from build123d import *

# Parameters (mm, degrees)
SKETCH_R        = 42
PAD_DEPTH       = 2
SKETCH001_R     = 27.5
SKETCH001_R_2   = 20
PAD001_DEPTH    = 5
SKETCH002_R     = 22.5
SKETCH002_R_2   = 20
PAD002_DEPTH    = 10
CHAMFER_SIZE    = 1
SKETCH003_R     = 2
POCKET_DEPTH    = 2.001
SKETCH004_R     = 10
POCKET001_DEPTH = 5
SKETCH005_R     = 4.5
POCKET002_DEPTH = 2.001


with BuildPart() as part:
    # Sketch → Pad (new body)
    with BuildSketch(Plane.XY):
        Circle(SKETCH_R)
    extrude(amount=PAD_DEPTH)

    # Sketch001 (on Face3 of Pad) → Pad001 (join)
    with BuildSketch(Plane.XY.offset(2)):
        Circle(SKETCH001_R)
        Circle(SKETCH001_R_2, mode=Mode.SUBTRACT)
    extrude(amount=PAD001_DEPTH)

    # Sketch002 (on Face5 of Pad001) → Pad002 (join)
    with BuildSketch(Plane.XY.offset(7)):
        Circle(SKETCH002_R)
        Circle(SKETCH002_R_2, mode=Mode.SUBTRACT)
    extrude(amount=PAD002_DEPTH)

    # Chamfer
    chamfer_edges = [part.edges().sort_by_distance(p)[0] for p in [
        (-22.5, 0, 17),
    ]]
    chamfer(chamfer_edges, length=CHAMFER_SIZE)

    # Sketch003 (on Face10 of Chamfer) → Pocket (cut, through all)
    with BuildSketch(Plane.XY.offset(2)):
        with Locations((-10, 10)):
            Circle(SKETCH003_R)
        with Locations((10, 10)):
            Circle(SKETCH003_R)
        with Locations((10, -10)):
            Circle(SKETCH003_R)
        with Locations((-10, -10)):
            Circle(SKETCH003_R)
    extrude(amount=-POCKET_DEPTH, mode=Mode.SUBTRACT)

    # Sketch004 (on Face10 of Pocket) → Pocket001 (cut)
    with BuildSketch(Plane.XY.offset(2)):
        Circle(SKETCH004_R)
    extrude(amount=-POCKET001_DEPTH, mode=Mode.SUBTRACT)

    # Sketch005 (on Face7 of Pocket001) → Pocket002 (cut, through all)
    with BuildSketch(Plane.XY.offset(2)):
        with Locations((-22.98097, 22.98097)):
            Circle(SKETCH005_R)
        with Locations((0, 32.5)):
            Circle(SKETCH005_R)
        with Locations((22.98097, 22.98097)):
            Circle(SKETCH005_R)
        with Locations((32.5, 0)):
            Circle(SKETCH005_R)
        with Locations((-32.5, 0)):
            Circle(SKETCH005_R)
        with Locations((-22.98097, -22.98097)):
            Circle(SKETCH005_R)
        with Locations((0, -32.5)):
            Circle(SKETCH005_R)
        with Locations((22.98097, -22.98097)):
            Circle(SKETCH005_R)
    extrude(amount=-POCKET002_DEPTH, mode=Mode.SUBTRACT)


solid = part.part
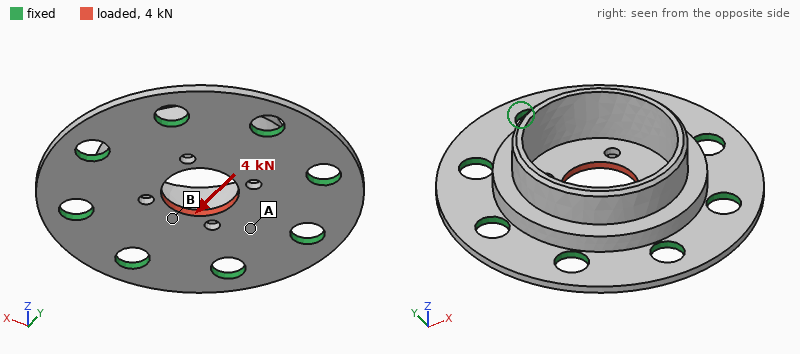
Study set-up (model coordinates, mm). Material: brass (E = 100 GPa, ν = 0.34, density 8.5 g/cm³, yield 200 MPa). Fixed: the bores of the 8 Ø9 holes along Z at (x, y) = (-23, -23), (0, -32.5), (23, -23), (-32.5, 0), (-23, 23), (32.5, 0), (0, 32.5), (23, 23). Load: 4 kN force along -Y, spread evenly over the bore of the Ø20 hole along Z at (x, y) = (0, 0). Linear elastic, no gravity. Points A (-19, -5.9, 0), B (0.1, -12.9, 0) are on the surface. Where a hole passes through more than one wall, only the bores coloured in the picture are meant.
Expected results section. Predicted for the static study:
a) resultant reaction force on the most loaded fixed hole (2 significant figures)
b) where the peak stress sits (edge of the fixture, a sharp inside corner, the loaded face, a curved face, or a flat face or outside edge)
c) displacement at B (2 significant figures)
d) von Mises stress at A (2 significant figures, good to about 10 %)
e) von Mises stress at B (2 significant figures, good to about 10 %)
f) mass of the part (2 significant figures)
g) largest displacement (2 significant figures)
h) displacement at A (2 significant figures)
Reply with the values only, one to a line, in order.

830 N
a curved face
4.8 µm
8.8 MPa
28 MPa
150 g
6.9 µm
1.4 µm
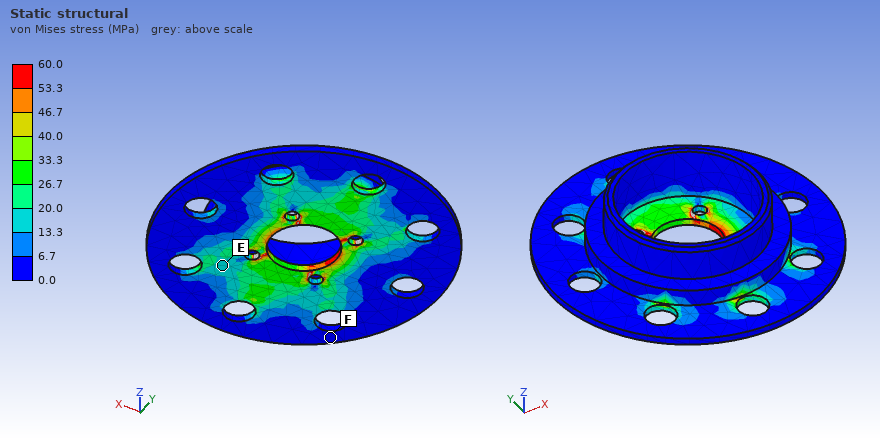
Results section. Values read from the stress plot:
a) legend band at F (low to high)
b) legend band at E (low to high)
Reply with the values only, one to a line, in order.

0.0 to 6.7 MPa
13.3 to 20.0 MPa
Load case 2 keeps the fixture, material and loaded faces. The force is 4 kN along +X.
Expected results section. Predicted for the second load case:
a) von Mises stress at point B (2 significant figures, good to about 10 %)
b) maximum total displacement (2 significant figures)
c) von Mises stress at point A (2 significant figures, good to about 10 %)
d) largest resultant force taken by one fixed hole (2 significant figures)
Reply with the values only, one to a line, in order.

33 MPa
6.9 µm
23 MPa
830 N
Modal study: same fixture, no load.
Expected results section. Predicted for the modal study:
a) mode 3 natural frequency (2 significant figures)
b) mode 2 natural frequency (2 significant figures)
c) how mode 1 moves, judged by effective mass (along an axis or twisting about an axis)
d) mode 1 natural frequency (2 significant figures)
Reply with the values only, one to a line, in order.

12 kHz
12 kHz
along Z
9800 Hz
